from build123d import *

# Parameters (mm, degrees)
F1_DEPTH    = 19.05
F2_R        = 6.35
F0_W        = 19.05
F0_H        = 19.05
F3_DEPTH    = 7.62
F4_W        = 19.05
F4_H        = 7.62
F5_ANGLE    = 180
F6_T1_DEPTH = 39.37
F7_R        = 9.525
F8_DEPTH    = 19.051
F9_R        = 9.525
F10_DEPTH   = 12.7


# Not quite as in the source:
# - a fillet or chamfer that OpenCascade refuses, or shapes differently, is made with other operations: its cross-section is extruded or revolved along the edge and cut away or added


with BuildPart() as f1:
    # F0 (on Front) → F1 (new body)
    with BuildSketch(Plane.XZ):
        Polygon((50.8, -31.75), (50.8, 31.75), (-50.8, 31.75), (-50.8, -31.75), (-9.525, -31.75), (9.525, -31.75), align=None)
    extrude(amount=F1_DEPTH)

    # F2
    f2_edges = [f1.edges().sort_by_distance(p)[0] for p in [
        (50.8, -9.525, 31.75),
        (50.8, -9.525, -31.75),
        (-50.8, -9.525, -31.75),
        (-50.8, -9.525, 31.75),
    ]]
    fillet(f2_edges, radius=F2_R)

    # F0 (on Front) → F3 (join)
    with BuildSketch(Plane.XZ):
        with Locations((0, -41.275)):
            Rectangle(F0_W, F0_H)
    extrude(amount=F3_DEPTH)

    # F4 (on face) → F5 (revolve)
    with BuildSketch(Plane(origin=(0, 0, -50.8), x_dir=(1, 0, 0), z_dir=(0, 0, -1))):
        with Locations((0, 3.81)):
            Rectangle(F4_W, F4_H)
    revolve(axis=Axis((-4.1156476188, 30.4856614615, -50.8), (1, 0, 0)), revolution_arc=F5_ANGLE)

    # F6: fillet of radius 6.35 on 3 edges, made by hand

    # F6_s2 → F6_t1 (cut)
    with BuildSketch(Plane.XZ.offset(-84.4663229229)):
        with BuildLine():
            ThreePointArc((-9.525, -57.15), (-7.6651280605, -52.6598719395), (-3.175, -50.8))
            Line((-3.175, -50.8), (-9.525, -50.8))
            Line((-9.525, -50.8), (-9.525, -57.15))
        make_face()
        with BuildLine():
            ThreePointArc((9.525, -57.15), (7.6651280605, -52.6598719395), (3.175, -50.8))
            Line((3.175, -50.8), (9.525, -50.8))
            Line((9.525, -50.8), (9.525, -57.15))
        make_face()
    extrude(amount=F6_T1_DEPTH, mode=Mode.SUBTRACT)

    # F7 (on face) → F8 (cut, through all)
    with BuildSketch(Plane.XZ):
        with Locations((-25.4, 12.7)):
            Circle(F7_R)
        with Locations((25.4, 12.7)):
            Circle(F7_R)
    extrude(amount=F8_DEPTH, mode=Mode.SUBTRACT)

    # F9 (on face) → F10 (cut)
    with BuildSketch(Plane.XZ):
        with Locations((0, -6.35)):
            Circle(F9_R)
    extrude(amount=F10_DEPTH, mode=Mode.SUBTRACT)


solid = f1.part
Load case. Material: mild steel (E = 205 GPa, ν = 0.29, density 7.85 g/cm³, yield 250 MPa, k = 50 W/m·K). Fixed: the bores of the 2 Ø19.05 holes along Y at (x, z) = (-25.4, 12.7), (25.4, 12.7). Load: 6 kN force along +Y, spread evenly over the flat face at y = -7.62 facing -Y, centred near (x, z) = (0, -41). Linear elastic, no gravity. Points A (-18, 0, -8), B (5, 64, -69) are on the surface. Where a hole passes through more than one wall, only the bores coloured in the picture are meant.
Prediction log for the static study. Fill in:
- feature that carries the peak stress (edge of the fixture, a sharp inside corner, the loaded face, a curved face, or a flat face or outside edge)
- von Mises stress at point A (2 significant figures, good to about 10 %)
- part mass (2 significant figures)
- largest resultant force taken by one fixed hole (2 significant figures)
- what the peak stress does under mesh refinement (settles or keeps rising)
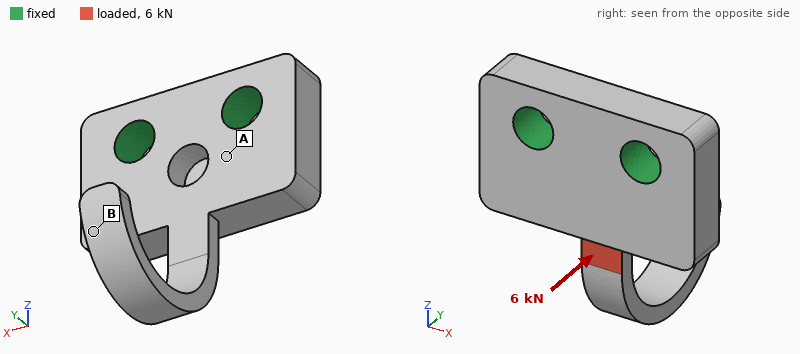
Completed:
a sharp inside corner
50 MPa
990 g
3.0 kN
keeps rising
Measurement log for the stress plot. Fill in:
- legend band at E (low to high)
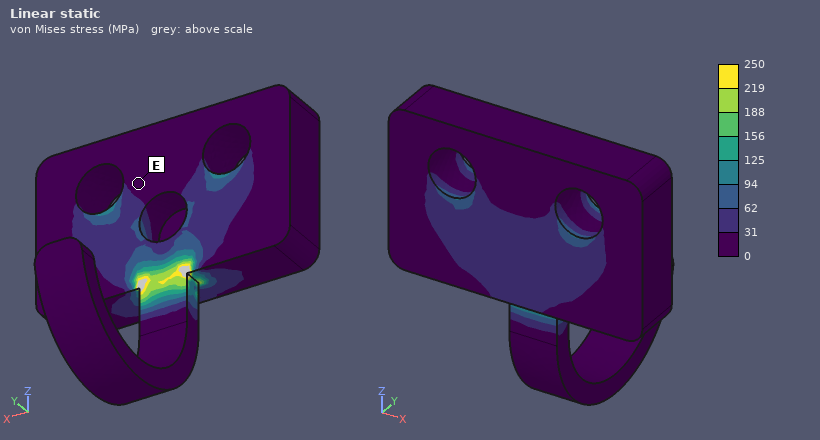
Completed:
0 to 31 MPa
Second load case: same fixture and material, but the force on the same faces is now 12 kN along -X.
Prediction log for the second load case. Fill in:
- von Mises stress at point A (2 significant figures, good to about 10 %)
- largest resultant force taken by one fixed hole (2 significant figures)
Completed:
31 MPa
11 kN
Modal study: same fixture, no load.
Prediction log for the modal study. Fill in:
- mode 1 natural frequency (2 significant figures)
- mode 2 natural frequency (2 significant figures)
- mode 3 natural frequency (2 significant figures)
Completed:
490 Hz
650 Hz
1300 Hz
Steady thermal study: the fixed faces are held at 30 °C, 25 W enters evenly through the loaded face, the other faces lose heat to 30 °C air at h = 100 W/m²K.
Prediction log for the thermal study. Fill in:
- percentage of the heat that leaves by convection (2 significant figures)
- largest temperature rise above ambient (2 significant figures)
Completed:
49 %
38 K
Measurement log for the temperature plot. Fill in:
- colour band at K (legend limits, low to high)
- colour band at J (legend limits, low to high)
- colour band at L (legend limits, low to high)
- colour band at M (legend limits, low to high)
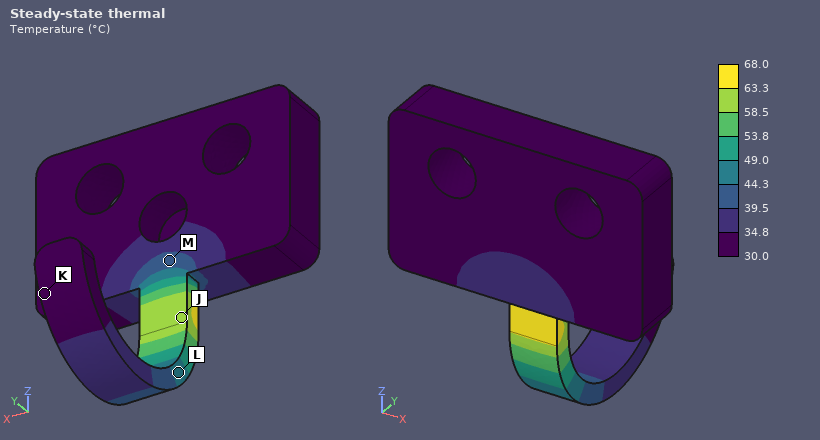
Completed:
30.0 to 34.8 °C
58.5 to 63.3 °C
44.3 to 49.0 °C
39.5 to 44.3 °C
